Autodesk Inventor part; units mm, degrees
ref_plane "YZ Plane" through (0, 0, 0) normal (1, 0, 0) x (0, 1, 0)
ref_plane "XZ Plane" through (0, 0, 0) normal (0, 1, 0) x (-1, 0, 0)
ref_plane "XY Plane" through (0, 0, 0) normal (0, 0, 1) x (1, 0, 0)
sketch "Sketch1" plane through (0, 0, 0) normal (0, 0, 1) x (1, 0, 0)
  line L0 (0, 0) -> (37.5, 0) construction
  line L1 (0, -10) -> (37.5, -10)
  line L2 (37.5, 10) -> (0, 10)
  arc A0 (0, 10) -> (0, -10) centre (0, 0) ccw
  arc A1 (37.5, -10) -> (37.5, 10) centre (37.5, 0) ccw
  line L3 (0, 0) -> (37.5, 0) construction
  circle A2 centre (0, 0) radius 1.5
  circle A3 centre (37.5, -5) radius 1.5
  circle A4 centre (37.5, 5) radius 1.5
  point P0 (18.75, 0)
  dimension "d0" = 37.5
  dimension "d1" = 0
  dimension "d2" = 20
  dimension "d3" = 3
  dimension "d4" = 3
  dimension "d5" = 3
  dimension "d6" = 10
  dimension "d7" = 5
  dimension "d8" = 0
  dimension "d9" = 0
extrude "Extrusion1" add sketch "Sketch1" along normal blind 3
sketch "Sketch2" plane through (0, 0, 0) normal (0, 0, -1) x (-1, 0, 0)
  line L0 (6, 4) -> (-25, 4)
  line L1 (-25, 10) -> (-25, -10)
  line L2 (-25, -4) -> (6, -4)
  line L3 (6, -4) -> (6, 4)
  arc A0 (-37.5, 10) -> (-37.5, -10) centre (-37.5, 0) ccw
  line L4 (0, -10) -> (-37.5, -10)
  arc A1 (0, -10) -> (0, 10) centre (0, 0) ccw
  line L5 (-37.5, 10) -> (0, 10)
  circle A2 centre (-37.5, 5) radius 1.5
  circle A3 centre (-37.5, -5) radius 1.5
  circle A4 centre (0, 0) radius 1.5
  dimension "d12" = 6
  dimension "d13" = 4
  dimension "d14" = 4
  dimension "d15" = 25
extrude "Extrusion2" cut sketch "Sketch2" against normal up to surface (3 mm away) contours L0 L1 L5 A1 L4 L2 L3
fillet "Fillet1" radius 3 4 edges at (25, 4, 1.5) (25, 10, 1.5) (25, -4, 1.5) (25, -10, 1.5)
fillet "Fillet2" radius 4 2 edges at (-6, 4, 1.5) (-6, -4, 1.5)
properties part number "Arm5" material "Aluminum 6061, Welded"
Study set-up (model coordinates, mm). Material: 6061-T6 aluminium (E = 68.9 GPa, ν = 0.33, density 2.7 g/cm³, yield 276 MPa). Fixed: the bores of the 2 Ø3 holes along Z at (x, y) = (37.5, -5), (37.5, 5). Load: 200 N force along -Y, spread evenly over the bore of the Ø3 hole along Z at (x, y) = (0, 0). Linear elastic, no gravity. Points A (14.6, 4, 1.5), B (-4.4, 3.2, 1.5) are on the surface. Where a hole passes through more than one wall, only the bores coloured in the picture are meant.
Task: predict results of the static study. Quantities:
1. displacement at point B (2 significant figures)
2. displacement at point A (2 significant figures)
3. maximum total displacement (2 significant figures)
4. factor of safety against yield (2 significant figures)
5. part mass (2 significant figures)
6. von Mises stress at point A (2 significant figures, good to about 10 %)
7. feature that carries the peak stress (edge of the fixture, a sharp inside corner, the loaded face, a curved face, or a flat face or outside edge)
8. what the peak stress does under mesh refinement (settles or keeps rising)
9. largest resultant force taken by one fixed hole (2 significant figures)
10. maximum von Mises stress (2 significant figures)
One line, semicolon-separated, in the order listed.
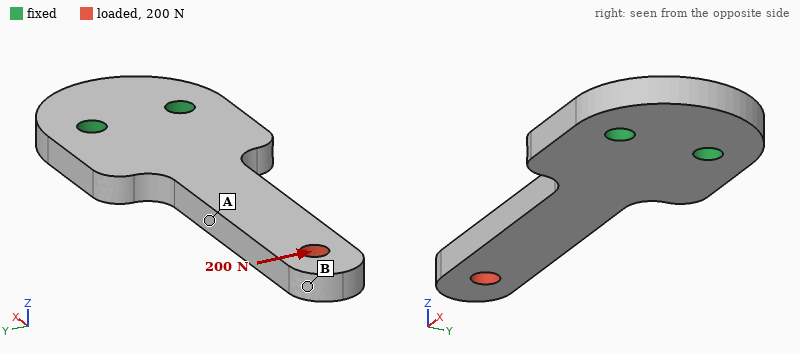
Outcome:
0.20 mm; 0.052 mm; 0.21 mm; 1.5; 5.1 g; 91 MPa; a curved face; settles; 640 N; 180 MPa
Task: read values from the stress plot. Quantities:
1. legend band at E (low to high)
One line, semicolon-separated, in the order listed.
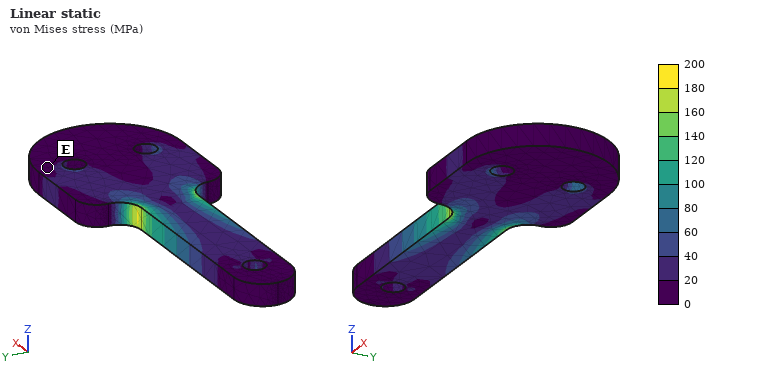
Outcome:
0 to 20 MPa
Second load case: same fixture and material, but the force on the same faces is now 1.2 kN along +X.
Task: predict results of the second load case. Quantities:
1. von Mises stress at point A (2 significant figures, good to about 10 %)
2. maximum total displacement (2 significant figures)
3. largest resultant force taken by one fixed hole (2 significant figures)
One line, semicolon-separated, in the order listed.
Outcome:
50 MPa; 26 µm; 620 N
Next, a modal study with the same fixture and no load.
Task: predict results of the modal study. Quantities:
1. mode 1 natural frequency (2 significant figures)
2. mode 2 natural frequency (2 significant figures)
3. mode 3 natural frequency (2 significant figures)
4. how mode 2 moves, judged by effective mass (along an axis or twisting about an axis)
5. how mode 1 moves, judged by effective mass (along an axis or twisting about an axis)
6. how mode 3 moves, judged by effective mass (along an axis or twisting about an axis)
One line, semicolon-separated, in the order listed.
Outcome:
1800 Hz; 6200 Hz; 9400 Hz; along Y; along Z; along Z
